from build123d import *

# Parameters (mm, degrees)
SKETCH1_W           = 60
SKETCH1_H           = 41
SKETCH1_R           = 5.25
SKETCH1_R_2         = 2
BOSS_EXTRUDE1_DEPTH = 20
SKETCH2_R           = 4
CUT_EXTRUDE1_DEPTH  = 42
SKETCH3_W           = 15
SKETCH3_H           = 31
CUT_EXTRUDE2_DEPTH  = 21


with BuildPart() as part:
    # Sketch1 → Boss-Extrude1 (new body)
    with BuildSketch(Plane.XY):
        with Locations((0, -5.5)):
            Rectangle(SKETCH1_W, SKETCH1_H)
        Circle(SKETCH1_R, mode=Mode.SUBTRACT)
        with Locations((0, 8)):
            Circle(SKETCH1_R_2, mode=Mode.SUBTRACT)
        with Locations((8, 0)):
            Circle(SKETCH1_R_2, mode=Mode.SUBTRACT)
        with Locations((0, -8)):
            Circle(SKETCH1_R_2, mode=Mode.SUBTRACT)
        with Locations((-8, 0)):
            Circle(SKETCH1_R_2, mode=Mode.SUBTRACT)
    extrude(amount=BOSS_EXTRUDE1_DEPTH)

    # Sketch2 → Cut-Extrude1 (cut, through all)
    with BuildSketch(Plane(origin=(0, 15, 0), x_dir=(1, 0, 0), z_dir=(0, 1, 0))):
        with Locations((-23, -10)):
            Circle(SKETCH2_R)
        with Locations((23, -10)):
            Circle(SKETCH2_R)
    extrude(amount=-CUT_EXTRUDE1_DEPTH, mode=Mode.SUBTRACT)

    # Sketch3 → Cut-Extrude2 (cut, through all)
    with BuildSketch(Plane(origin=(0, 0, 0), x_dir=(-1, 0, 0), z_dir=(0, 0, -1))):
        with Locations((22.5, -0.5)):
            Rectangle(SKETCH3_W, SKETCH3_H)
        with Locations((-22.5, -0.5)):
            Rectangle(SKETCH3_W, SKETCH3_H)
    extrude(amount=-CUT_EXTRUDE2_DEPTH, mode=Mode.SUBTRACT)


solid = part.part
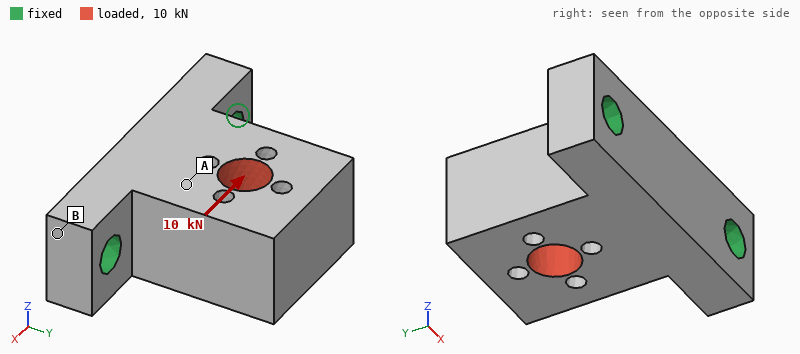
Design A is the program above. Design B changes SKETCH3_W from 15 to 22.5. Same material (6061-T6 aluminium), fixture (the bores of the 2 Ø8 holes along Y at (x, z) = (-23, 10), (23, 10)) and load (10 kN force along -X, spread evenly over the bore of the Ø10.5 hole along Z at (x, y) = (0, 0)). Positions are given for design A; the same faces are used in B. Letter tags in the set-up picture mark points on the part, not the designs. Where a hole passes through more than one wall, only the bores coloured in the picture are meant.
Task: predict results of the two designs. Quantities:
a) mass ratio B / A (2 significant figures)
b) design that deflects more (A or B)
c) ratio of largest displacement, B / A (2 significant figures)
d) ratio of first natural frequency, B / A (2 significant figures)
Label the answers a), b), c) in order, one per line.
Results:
a) 0.83
b) B
c) 2.2
d) 0.99
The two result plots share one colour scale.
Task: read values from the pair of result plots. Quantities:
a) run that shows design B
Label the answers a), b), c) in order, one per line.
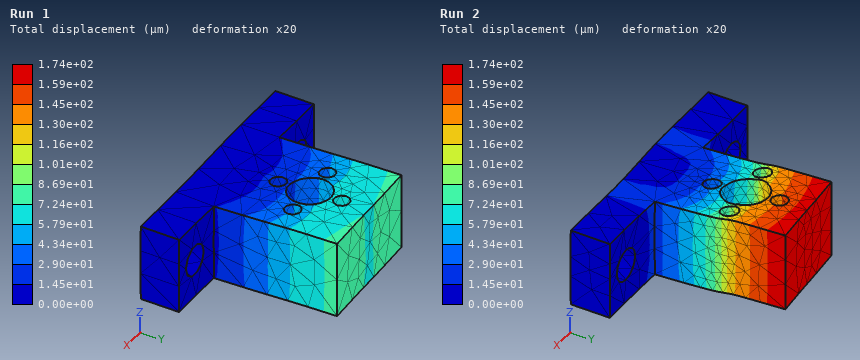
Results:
a) Run 2
